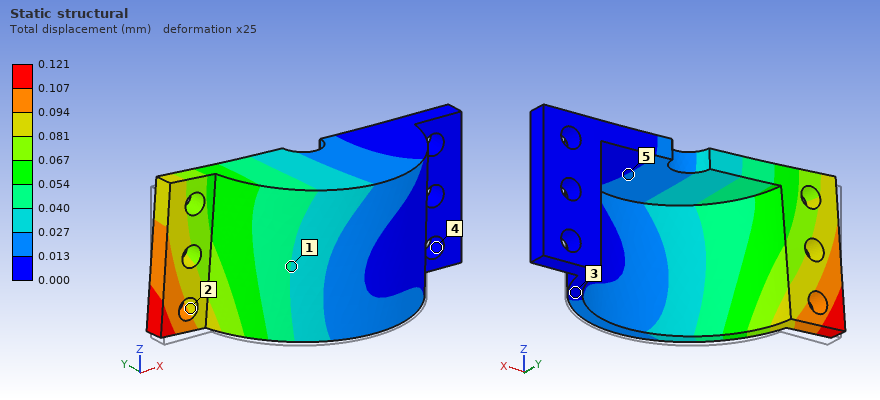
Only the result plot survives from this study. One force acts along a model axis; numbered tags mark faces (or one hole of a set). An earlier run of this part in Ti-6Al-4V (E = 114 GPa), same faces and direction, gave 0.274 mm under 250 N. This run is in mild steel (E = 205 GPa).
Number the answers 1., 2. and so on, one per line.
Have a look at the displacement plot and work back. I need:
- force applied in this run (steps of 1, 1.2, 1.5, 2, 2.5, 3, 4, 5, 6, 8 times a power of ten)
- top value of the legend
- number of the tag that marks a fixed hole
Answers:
1. 200 N
2. 0.121 mm
3. 4
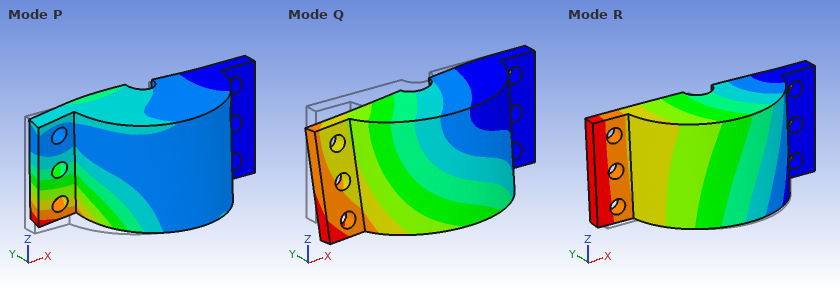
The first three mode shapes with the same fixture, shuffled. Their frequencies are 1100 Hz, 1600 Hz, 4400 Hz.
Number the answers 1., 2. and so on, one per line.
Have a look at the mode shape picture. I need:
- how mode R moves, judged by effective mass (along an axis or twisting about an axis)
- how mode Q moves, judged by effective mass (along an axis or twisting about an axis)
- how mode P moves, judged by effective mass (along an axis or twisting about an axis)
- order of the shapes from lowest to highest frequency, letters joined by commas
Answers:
1. along Y
2. along Z
3. along X
4. R, Q, P
